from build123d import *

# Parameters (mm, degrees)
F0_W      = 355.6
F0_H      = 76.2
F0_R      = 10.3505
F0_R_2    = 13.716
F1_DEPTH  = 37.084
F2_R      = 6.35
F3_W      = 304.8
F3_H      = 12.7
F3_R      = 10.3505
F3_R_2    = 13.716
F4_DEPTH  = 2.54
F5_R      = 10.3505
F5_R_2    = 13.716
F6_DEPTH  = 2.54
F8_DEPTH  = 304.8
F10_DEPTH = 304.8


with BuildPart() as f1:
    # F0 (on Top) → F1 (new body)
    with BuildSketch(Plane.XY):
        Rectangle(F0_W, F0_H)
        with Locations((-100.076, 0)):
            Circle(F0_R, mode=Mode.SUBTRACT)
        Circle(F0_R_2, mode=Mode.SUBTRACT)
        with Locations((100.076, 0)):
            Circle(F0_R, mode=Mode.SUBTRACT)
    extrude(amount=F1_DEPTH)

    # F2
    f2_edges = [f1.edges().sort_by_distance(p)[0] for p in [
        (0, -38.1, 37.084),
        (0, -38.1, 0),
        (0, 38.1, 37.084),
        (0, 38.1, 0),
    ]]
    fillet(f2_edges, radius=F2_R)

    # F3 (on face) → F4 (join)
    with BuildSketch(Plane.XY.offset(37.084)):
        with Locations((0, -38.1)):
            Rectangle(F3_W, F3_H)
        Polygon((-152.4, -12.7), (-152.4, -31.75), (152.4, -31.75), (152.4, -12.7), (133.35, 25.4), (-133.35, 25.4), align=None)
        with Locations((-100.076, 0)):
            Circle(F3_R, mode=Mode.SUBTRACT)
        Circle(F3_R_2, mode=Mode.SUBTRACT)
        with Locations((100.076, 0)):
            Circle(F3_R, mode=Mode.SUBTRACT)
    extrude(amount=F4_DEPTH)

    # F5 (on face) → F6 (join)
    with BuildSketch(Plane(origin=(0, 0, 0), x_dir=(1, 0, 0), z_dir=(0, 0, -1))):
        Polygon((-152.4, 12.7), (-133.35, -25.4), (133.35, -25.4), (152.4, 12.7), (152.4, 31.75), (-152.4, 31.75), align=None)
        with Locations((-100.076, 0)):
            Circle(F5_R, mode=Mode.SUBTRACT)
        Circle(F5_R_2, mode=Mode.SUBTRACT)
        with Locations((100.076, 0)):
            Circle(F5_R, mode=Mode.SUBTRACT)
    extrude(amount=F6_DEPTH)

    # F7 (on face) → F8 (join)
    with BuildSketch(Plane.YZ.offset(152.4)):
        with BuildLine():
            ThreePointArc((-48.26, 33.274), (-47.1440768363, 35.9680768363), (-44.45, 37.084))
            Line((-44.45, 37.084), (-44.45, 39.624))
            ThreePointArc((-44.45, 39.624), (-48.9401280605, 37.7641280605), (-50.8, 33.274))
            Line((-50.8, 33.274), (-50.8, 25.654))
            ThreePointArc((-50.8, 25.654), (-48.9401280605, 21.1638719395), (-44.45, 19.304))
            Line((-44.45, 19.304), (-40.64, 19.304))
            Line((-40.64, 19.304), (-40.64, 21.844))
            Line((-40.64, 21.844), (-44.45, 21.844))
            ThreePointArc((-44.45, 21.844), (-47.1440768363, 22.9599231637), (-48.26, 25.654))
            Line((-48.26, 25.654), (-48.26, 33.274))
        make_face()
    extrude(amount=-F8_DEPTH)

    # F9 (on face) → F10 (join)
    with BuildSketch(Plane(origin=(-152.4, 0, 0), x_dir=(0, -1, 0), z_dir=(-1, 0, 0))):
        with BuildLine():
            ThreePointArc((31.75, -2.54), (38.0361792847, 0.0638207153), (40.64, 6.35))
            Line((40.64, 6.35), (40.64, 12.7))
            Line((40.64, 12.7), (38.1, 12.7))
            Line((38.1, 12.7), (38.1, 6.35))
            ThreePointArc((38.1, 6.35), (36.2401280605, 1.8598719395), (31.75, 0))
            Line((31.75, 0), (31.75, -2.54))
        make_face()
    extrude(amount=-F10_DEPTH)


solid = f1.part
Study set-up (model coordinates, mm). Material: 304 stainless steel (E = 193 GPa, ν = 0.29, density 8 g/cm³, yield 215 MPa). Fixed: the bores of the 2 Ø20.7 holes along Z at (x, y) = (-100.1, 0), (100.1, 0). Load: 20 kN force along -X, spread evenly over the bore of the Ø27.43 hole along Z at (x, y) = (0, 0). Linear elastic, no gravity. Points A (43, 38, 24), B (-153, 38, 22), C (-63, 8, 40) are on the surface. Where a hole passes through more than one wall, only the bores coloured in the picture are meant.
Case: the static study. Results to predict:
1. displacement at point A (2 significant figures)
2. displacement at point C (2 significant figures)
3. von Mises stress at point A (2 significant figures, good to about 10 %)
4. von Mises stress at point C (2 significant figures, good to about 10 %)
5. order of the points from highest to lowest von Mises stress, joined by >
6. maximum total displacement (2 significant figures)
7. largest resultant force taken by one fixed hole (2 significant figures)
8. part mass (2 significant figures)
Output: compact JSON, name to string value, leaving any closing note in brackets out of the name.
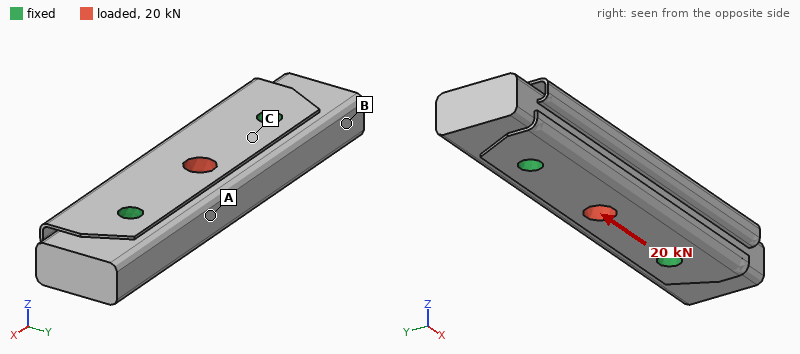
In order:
{"displacement at point A": "1.1 µm", "displacement at point C": "0.69 µm", "von Mises stress at point A": "2.4 MPa", "von Mises stress at point C": "4.2 MPa", "order of the points from highest to lowest von Mises stress, joined by >": "C > A > B", "maximum total displacement": "2.0 µm", "largest resultant force taken by one fixed hole": "10 kN", "part mass": "8.6 kg"}
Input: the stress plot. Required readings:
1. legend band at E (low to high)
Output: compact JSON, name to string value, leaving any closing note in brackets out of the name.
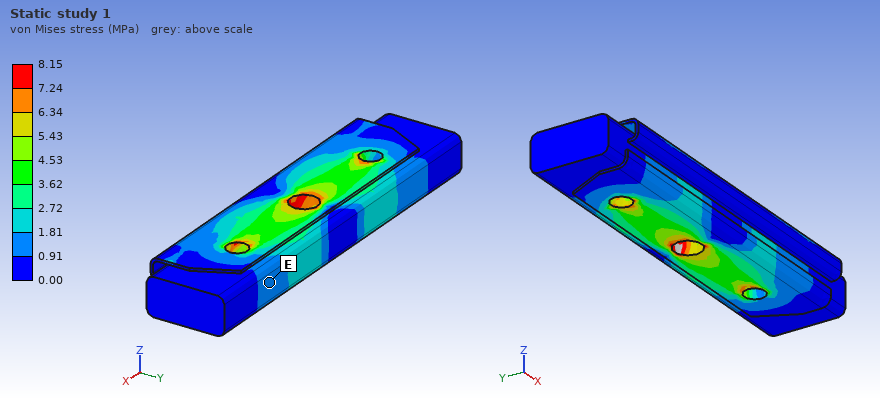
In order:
{"legend band at E": "0.91 to 1.81 MPa"}
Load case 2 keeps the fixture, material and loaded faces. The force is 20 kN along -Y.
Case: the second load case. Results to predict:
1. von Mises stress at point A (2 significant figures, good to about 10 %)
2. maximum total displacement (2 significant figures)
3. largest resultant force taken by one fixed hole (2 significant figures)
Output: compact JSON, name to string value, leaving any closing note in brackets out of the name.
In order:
{"von Mises stress at point A": "6.0 MPa", "maximum total displacement": "14 µm", "largest resultant force taken by one fixed hole": "10 kN"}
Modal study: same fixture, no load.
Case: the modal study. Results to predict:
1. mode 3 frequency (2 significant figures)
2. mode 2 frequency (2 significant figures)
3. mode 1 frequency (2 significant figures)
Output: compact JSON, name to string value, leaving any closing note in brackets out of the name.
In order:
{"mode 3 frequency": "2700 Hz", "mode 2 frequency": "1800 Hz", "mode 1 frequency": "1800 Hz"}
